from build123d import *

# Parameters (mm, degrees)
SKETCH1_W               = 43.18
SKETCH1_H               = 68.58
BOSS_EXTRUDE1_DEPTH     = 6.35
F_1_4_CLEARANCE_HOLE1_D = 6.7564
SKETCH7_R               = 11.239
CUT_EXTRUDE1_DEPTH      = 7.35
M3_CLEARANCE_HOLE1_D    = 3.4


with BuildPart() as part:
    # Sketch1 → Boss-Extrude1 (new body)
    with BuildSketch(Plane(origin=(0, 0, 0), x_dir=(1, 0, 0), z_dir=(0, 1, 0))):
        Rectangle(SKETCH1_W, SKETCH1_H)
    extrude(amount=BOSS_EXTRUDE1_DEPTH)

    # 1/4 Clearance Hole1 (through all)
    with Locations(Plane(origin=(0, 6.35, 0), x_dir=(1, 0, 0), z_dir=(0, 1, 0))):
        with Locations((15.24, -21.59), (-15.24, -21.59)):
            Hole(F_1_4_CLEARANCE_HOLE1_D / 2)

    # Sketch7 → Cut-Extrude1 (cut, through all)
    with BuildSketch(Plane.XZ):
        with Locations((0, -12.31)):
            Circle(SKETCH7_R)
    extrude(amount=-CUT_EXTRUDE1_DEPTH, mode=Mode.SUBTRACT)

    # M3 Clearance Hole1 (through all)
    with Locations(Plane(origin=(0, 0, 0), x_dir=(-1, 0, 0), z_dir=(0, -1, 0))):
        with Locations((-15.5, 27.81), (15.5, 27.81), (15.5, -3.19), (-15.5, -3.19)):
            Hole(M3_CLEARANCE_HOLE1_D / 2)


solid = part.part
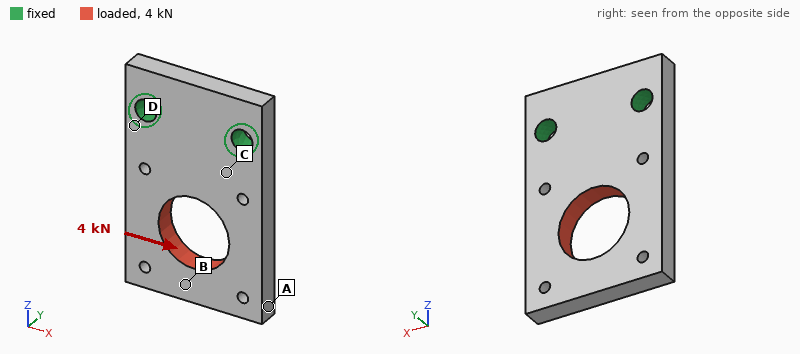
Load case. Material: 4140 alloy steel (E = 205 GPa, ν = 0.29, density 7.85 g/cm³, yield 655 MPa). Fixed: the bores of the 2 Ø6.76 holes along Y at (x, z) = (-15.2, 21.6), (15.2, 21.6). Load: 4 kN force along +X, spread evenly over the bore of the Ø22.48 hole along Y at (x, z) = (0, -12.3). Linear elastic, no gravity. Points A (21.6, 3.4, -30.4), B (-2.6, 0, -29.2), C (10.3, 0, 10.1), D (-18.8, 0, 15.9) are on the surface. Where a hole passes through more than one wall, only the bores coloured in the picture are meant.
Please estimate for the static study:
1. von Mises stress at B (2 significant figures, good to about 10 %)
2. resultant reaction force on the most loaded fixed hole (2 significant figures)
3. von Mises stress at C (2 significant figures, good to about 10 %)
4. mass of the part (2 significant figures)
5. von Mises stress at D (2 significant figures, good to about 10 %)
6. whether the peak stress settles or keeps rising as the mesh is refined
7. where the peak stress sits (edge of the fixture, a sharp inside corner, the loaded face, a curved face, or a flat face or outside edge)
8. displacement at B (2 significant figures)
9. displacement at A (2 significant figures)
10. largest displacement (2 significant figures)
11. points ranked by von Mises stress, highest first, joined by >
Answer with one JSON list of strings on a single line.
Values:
["19 MPa", "4.4 kN", "32 MPa", "120 g", "53 MPa", "keeps rising", "edge of the fixture", "29 µm", "31 µm", "33 µm", "D > C > B > A"]
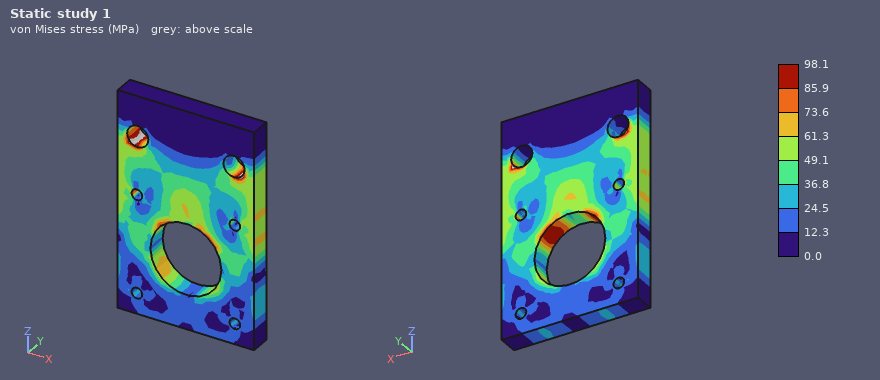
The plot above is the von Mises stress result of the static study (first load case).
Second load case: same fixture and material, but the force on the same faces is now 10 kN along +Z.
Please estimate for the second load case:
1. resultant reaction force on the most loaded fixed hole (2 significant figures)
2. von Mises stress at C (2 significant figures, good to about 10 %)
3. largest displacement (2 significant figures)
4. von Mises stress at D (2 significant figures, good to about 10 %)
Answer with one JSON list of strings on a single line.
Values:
["5.0 kN", "41 MPa", "16 µm", "49 MPa"]
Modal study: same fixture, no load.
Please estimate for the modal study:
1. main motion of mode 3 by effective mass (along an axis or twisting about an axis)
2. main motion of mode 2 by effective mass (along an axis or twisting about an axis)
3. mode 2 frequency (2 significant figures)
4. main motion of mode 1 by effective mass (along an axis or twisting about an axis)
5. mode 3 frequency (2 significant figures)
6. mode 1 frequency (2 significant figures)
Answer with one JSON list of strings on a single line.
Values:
["along X", "twisting about Z", "4400 Hz", "along Y", "7400 Hz", "1700 Hz"]
